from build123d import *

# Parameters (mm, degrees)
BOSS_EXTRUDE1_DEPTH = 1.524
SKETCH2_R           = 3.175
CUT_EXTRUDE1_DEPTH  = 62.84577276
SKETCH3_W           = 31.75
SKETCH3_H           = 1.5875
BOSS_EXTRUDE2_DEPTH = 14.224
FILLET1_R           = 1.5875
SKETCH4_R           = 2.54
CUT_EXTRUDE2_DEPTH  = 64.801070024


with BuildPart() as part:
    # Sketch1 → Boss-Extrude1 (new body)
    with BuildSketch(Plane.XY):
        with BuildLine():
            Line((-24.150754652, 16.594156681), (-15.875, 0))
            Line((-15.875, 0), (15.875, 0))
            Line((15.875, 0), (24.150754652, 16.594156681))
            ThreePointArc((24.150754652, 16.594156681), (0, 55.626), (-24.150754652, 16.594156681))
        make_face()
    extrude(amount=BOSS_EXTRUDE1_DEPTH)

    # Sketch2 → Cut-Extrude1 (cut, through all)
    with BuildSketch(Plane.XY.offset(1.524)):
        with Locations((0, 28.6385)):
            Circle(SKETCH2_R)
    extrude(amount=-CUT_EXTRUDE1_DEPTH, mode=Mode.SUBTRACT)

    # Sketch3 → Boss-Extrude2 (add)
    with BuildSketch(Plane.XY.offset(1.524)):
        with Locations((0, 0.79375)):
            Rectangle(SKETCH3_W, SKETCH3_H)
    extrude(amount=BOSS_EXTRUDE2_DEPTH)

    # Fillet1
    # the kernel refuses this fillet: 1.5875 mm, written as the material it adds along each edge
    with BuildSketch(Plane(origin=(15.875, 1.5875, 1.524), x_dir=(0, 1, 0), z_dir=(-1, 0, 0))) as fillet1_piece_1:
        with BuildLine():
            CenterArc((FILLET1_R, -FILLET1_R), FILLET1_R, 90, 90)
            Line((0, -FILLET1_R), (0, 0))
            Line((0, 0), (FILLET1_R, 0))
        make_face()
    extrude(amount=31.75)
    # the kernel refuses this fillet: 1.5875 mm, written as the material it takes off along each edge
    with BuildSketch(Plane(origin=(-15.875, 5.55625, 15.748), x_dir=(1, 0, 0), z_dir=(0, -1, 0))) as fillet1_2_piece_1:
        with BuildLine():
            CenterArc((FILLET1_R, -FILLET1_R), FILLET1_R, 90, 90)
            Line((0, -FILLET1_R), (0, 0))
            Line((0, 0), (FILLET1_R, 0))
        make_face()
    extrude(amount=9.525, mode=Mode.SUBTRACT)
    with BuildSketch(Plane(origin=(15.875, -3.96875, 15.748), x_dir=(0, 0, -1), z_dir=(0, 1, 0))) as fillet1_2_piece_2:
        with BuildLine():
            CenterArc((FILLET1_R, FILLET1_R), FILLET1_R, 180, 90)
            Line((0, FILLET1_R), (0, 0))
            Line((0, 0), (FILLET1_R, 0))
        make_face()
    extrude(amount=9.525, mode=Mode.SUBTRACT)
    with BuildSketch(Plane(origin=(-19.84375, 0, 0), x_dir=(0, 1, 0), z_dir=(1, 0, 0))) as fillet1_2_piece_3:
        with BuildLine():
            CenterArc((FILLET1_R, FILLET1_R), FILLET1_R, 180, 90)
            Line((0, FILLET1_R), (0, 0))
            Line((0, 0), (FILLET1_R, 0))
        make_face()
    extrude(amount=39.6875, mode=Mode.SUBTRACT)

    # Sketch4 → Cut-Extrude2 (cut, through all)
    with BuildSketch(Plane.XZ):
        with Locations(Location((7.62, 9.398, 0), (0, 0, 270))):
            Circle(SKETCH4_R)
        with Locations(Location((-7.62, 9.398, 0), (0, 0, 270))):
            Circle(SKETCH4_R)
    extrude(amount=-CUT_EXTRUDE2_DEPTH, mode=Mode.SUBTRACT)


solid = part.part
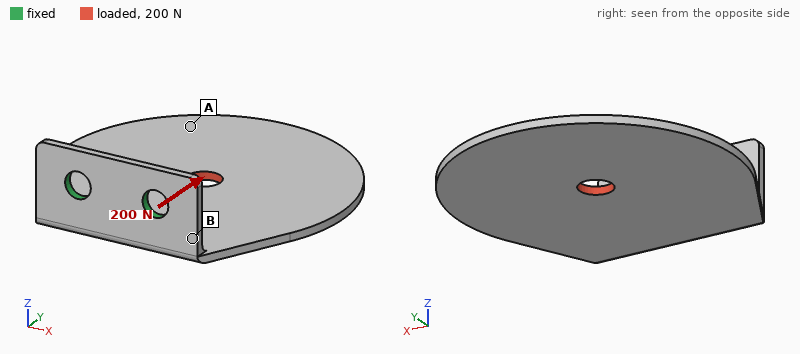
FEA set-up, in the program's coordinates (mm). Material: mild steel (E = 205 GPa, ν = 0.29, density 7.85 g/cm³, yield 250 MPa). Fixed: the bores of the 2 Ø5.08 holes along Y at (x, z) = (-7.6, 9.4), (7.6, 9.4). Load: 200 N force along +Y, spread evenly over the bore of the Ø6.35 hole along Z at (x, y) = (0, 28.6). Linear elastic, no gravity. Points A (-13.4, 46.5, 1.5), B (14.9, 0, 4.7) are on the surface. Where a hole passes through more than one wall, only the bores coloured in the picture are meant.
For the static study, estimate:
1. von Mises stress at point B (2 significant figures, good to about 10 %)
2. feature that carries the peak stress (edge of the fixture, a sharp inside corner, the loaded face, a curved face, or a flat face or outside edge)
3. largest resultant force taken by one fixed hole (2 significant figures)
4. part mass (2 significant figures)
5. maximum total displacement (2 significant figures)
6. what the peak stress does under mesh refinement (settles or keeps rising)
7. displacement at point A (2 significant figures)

41 MPa
edge of the fixture
100 N
34 g
0.12 mm
keeps rising
0.10 mm
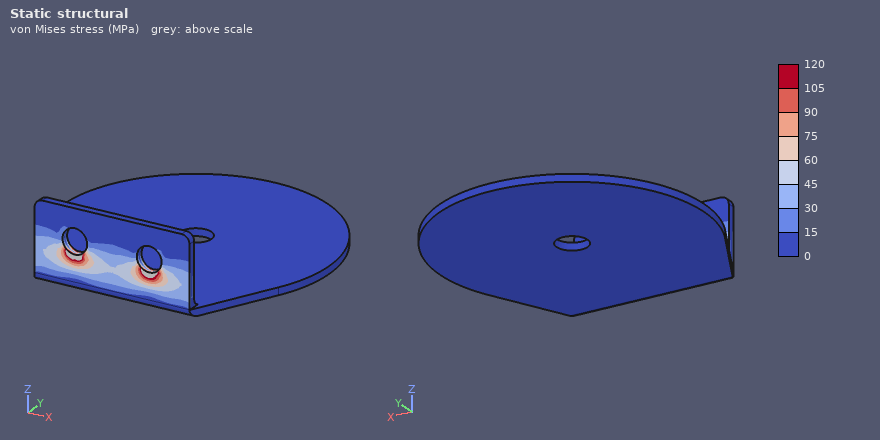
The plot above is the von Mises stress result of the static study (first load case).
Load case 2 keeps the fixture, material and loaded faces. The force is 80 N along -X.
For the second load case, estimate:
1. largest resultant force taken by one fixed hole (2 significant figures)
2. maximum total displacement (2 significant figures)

130 N
51 µm
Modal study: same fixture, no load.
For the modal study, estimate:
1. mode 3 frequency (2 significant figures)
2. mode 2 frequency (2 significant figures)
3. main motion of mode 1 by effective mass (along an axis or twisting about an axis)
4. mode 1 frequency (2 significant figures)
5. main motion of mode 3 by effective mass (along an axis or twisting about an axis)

1500 Hz
1000 Hz
along Z
370 Hz
along X
